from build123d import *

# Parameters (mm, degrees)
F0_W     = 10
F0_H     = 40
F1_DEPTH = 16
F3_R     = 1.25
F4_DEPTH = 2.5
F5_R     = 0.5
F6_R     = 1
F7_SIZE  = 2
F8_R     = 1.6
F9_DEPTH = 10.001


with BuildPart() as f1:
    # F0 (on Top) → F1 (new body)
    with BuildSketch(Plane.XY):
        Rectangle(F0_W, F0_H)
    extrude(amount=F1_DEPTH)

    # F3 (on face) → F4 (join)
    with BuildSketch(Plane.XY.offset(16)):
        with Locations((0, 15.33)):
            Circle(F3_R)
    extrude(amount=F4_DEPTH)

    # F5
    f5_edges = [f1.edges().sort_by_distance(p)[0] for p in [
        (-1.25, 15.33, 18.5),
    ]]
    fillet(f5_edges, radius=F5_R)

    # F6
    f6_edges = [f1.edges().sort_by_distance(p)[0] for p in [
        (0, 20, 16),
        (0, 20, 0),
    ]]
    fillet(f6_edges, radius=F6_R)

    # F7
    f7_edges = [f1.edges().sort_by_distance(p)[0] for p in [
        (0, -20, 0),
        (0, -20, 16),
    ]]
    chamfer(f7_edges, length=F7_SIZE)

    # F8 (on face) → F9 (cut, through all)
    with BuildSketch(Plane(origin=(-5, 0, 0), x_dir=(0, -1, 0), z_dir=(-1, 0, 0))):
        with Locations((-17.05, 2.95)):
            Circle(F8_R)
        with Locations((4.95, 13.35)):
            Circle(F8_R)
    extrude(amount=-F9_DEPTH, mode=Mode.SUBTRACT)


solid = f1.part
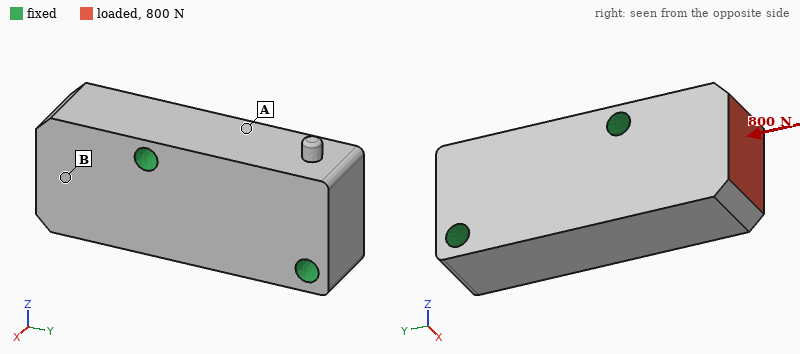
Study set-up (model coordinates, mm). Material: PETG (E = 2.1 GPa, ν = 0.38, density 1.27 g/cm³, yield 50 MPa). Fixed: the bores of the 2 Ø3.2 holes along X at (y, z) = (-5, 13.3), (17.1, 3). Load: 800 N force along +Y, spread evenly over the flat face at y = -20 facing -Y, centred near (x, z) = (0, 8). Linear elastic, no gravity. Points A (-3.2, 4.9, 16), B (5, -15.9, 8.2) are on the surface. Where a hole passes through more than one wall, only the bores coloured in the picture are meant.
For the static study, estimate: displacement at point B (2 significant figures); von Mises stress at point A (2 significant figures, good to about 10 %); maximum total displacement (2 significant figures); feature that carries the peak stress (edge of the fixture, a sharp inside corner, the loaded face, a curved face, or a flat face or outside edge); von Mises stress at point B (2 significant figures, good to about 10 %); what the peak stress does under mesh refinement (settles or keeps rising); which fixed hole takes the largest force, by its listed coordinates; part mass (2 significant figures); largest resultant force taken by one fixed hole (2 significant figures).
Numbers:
69 µm
2.6 MPa
99 µm
edge of the fixture
6.8 MPa
keeps rising
(-5, 13.3)
7.9 g
570 N
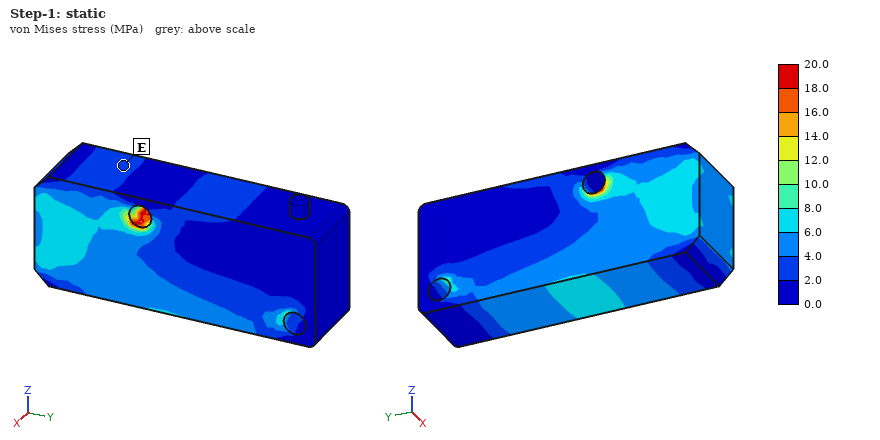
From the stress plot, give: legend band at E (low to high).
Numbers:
2.0 to 4.0 MPa
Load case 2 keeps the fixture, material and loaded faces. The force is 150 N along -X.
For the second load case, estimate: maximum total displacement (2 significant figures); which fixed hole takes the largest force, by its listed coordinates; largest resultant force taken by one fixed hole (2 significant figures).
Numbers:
0.13 mm
(-5, 13.3)
180 N
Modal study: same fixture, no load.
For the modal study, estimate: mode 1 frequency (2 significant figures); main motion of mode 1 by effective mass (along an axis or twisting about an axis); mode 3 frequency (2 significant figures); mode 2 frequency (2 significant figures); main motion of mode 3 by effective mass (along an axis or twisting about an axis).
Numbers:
5300 Hz
along X
8300 Hz
6400 Hz
twisting about Y
